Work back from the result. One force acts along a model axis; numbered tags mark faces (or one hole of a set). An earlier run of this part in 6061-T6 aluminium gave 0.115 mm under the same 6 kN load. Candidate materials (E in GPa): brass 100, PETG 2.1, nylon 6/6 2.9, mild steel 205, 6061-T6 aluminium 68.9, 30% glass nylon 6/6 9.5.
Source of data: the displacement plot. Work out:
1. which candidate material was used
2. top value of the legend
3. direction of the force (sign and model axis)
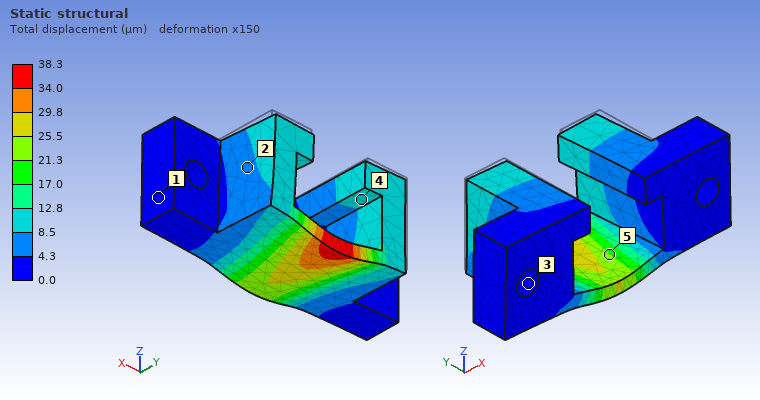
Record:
mild steel
38.3 µm
-Z
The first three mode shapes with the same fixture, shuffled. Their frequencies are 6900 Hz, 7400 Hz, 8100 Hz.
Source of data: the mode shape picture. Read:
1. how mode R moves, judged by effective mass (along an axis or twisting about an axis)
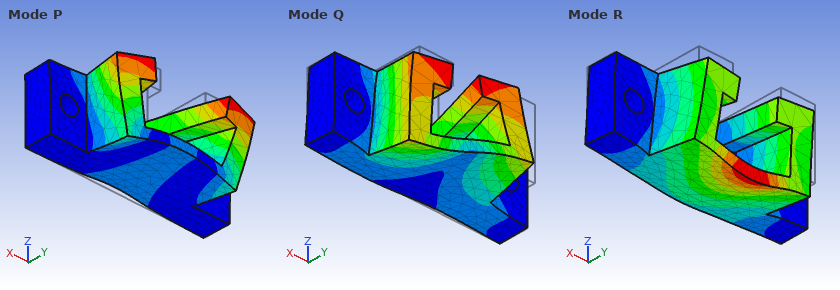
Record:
along Z
